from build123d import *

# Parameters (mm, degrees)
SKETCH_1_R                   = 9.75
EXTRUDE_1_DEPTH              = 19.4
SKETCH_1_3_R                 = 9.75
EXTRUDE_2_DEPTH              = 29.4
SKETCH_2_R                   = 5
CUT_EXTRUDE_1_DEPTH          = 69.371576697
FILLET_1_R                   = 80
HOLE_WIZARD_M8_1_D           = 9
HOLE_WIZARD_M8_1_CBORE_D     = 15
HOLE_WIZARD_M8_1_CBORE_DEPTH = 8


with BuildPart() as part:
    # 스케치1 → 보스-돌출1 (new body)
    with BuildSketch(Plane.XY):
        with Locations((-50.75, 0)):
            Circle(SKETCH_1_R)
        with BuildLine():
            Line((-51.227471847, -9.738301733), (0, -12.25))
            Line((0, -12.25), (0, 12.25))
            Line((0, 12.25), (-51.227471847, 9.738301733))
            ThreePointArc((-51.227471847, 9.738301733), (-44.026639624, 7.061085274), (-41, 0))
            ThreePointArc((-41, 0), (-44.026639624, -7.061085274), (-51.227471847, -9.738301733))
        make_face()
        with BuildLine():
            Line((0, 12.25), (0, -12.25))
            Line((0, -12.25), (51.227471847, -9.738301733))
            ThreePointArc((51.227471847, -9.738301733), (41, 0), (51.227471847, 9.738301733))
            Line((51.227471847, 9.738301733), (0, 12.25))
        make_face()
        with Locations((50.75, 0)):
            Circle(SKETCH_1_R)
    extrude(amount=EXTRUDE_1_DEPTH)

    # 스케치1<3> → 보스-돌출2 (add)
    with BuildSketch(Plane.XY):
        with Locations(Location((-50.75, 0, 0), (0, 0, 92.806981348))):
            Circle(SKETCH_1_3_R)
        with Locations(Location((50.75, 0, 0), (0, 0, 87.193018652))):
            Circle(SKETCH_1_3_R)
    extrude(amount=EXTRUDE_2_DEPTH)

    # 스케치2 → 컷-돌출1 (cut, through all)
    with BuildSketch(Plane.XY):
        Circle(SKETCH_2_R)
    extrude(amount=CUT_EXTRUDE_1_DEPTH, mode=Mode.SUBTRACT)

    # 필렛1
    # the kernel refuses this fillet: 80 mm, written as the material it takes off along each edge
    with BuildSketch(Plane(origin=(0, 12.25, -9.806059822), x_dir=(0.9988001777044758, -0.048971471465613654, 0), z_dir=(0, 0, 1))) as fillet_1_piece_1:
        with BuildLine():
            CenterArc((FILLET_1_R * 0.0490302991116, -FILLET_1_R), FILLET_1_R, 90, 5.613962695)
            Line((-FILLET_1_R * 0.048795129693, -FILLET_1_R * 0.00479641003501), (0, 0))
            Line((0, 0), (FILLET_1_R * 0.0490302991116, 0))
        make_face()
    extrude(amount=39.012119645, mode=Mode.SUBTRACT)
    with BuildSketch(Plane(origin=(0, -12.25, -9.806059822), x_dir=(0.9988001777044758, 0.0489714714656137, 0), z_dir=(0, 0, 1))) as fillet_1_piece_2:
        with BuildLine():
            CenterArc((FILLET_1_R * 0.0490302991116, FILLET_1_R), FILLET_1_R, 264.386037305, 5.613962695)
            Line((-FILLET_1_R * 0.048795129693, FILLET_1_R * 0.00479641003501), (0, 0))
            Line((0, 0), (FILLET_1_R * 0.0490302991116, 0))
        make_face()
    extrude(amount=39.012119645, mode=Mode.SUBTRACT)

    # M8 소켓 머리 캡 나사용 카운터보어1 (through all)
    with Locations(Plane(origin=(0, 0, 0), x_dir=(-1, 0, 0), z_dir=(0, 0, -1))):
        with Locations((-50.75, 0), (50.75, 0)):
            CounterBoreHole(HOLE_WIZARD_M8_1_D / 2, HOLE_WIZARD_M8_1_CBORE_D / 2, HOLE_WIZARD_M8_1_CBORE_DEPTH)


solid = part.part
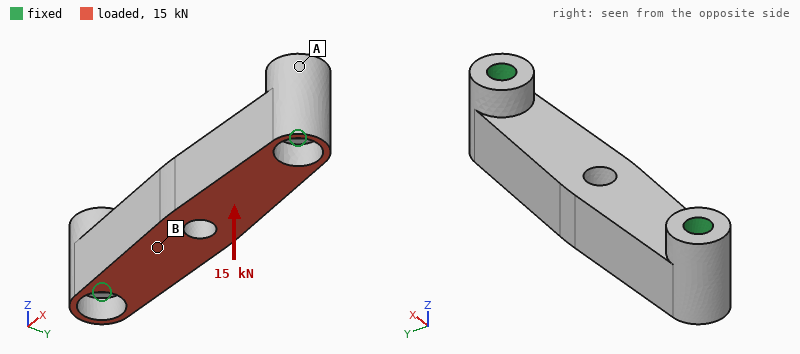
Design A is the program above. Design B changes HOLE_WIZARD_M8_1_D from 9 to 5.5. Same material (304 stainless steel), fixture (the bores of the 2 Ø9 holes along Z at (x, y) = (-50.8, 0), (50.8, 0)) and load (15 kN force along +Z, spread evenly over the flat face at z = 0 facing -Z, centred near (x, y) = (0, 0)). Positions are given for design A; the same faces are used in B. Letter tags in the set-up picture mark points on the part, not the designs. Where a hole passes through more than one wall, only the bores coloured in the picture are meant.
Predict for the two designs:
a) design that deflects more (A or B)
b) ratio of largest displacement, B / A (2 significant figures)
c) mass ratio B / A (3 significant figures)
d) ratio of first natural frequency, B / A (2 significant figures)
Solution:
B
1.1
1.04
0.90
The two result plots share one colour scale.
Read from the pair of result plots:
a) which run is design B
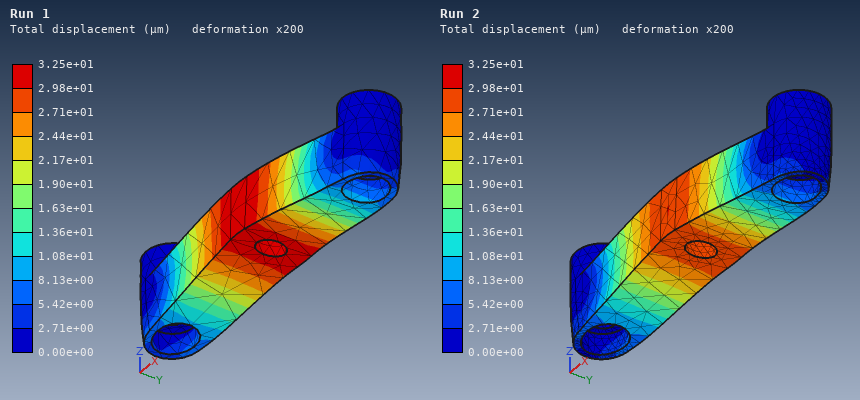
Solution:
Run 1
